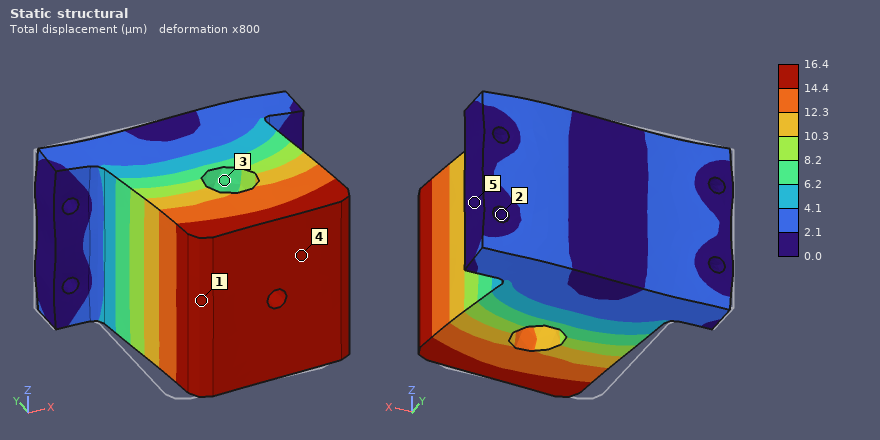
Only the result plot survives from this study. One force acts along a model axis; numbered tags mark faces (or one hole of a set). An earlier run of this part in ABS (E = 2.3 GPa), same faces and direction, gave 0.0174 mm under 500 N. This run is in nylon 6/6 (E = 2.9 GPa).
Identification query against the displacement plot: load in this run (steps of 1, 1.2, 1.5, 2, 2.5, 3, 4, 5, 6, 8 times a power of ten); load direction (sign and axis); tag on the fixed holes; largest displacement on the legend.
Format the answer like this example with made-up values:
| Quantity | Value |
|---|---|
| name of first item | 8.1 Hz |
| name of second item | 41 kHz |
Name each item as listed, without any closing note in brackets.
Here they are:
| Quantity | Value |
|---|---|
| load in this run | 600 N |
| load direction | +X |
| tag on the fixed holes | 2 |
| largest displacement on the legend | 16.4 µm |
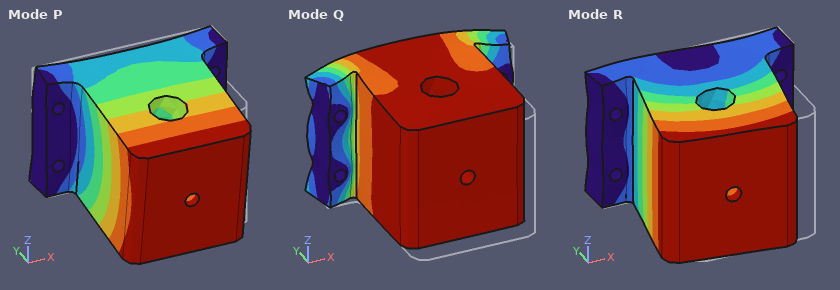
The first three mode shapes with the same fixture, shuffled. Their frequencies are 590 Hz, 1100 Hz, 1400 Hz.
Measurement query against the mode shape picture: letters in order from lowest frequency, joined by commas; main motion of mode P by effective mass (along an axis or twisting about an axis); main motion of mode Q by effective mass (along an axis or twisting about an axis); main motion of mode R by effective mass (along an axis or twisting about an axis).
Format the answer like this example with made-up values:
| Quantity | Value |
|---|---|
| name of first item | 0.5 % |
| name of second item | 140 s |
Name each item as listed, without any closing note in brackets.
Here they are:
| Quantity | Value |
|---|---|
| letters in order from lowest frequency, joined by commas | P, R, Q |
| main motion of mode P by effective mass | along Z |
| main motion of mode Q by effective mass | along Y |
| main motion of mode R by effective mass | along X |
